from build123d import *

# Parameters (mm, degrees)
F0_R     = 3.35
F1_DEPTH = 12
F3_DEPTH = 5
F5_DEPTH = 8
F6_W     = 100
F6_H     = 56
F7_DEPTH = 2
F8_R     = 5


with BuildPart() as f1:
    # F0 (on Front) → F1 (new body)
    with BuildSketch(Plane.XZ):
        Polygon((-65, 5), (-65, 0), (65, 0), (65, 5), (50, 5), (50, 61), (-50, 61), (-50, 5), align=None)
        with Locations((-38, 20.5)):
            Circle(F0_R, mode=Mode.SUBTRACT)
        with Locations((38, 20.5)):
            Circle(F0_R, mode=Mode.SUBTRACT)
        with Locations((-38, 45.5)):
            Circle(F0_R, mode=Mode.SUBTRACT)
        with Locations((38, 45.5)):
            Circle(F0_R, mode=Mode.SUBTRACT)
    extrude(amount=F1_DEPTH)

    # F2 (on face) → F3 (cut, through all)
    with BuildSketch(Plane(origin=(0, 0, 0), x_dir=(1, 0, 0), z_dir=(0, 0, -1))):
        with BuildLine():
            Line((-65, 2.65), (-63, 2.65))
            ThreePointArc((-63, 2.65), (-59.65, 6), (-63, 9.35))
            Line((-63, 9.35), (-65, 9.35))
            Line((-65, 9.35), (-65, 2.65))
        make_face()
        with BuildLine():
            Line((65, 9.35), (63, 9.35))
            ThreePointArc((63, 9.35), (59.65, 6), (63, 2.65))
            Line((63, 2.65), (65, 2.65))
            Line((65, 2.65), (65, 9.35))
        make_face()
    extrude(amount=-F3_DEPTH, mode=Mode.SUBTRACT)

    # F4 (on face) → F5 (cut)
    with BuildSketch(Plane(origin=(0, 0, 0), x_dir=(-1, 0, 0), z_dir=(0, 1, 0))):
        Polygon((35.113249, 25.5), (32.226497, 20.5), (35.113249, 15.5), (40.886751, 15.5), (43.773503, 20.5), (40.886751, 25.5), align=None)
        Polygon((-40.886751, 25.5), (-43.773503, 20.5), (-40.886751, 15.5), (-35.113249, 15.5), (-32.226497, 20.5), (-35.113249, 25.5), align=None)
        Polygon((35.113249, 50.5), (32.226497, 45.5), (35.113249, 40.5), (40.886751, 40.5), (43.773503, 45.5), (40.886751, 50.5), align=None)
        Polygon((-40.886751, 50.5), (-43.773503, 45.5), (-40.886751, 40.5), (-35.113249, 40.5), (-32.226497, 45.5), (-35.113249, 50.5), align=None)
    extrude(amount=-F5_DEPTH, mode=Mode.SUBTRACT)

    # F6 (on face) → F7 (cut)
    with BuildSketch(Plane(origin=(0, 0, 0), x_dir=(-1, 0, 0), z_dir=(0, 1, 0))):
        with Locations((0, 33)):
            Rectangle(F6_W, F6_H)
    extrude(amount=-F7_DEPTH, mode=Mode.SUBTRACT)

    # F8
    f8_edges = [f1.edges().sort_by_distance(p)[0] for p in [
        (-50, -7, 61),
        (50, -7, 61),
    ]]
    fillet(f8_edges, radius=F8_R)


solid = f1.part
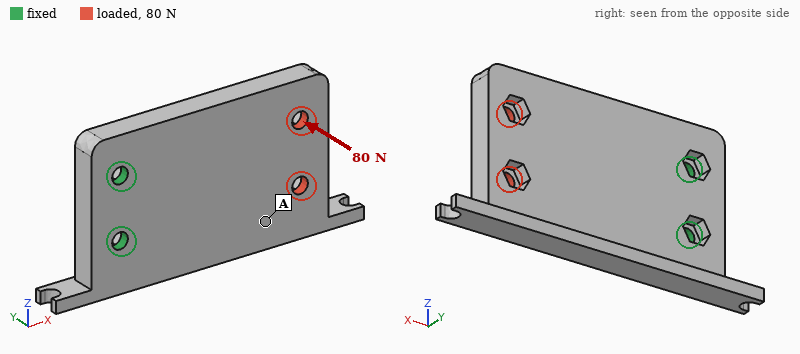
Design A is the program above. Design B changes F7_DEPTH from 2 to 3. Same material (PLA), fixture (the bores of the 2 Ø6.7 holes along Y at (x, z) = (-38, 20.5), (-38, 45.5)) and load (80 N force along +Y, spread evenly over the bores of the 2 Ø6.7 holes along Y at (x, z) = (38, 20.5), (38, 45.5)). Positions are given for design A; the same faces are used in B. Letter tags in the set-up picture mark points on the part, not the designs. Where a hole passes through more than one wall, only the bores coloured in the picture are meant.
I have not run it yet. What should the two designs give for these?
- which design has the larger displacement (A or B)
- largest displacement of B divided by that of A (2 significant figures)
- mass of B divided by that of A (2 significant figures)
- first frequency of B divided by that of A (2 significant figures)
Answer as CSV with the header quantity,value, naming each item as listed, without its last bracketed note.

quantity,value
which design has the larger displacement,B
largest displacement of B divided by that of A,1.2
mass of B divided by that of A,0.91
first frequency of B divided by that of A,0.97
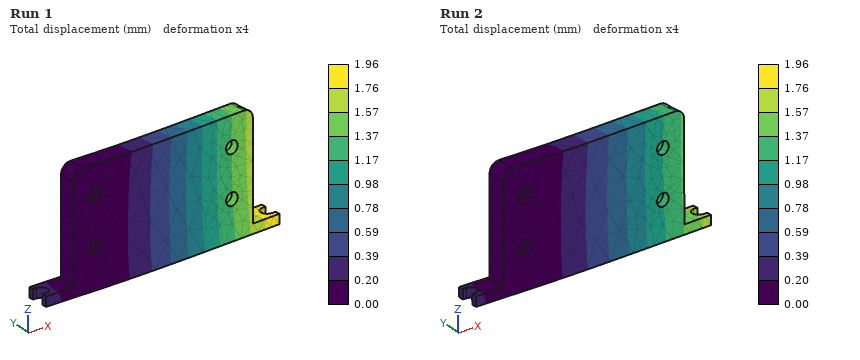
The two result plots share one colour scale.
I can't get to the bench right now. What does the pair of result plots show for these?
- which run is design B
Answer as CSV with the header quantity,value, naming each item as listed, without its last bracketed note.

quantity,value
which run is design B,Run 1
